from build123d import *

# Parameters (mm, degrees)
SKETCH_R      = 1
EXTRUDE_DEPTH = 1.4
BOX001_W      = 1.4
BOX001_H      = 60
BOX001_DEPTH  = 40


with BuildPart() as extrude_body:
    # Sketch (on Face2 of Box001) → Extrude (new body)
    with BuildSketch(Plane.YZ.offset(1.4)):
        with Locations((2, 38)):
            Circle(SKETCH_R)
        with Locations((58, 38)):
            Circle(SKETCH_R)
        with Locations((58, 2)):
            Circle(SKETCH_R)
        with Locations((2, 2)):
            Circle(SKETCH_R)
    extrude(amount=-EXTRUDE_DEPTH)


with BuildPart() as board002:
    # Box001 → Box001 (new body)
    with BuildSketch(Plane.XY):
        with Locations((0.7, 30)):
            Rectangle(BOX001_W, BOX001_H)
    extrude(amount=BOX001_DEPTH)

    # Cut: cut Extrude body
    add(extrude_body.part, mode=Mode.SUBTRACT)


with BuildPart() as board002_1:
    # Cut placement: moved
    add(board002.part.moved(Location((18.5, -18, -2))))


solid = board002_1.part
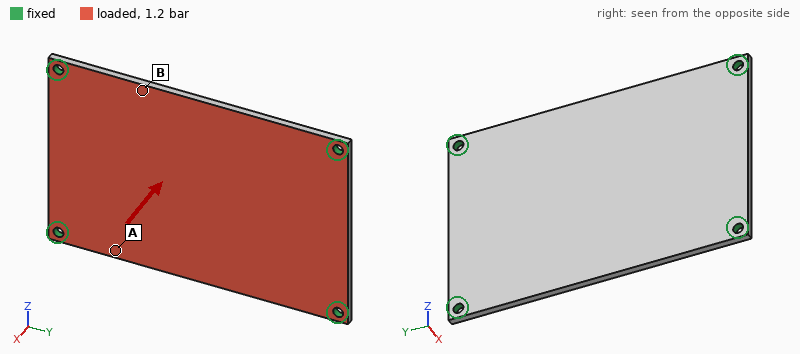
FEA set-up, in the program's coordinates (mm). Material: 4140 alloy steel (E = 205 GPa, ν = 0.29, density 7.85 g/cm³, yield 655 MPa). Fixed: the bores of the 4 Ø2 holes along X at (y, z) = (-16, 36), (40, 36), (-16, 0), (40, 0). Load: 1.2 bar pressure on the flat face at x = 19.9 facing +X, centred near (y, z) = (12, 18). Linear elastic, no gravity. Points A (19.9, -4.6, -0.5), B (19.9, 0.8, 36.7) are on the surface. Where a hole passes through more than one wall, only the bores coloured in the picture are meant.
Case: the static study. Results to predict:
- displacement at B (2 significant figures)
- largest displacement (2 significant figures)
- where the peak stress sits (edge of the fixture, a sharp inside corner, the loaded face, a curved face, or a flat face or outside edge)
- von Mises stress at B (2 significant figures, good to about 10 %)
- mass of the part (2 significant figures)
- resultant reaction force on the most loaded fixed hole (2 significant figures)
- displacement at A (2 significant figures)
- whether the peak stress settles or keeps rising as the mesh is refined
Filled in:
0.073 mm
0.11 mm
edge of the fixture
47 MPa
26 g
72 N
0.045 mm
keeps rising
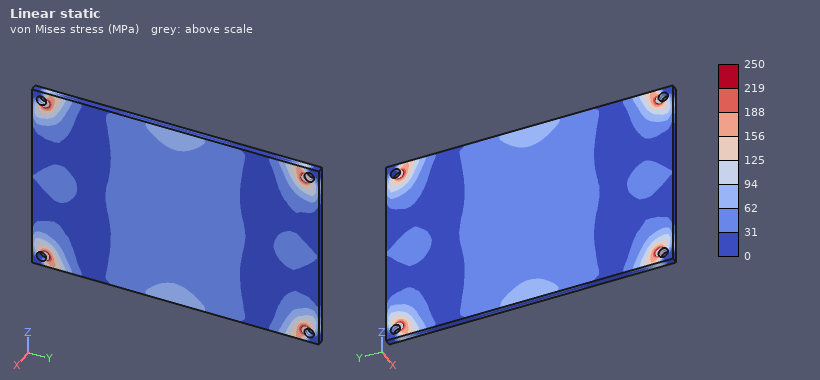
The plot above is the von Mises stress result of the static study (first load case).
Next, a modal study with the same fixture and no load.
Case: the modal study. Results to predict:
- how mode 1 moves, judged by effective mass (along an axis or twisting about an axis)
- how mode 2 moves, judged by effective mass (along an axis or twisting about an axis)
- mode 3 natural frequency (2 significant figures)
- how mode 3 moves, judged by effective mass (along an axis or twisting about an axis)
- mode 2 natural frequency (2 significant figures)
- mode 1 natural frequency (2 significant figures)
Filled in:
along X
twisting about Y
4600 Hz
twisting about Z
3200 Hz
1800 Hz
